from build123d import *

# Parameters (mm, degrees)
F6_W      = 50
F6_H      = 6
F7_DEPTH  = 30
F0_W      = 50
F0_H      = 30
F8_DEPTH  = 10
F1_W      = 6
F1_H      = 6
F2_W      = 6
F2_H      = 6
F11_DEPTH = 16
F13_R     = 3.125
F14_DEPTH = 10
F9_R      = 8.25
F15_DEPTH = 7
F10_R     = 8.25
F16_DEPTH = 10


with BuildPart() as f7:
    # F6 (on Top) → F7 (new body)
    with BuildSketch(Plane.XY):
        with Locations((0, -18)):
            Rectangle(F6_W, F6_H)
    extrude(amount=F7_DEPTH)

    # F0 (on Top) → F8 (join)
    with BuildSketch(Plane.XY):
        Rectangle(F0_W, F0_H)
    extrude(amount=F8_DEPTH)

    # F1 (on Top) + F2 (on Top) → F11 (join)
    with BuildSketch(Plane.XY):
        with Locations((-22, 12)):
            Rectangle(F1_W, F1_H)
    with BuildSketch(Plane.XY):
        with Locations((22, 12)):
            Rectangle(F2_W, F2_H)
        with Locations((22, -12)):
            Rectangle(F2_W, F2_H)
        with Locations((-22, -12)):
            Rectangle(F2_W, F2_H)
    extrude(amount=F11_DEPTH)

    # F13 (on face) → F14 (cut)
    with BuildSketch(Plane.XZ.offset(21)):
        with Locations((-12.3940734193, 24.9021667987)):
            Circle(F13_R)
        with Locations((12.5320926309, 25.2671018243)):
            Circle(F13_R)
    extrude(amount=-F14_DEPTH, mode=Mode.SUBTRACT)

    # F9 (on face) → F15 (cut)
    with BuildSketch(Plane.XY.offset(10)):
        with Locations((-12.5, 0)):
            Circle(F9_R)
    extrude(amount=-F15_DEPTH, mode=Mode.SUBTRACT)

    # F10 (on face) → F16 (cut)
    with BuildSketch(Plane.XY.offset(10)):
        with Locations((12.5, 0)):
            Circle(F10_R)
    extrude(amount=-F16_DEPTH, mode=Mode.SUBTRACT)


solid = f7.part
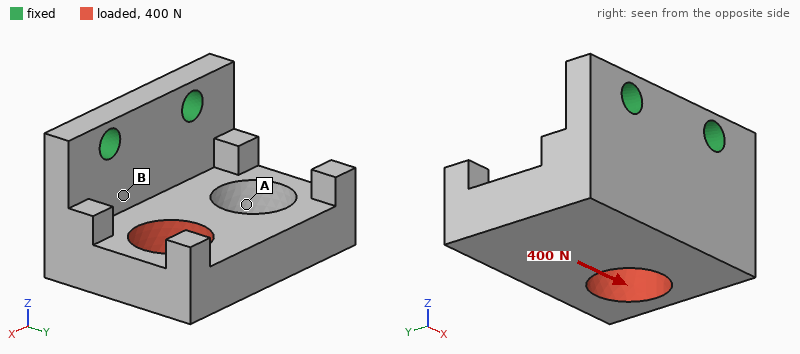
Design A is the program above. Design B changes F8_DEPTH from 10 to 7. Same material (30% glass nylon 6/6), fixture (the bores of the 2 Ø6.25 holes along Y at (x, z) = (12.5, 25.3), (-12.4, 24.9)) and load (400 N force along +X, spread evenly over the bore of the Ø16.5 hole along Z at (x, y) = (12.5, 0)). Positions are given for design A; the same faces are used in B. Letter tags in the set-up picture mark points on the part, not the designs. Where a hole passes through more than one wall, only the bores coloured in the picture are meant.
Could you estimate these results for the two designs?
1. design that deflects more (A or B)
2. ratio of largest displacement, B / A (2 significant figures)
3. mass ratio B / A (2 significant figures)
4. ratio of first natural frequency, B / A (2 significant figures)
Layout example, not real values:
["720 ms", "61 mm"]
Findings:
["B", "1.5", "0.87", "1.0"]
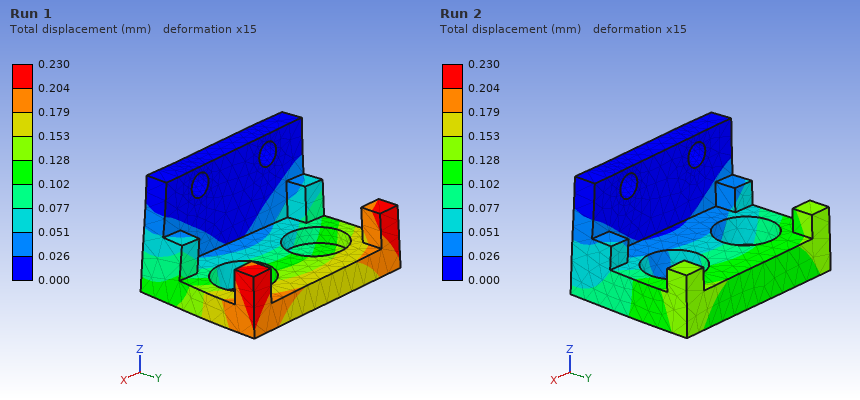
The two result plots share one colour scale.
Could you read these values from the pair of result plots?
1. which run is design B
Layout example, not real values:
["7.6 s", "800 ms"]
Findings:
["Run 1"]
